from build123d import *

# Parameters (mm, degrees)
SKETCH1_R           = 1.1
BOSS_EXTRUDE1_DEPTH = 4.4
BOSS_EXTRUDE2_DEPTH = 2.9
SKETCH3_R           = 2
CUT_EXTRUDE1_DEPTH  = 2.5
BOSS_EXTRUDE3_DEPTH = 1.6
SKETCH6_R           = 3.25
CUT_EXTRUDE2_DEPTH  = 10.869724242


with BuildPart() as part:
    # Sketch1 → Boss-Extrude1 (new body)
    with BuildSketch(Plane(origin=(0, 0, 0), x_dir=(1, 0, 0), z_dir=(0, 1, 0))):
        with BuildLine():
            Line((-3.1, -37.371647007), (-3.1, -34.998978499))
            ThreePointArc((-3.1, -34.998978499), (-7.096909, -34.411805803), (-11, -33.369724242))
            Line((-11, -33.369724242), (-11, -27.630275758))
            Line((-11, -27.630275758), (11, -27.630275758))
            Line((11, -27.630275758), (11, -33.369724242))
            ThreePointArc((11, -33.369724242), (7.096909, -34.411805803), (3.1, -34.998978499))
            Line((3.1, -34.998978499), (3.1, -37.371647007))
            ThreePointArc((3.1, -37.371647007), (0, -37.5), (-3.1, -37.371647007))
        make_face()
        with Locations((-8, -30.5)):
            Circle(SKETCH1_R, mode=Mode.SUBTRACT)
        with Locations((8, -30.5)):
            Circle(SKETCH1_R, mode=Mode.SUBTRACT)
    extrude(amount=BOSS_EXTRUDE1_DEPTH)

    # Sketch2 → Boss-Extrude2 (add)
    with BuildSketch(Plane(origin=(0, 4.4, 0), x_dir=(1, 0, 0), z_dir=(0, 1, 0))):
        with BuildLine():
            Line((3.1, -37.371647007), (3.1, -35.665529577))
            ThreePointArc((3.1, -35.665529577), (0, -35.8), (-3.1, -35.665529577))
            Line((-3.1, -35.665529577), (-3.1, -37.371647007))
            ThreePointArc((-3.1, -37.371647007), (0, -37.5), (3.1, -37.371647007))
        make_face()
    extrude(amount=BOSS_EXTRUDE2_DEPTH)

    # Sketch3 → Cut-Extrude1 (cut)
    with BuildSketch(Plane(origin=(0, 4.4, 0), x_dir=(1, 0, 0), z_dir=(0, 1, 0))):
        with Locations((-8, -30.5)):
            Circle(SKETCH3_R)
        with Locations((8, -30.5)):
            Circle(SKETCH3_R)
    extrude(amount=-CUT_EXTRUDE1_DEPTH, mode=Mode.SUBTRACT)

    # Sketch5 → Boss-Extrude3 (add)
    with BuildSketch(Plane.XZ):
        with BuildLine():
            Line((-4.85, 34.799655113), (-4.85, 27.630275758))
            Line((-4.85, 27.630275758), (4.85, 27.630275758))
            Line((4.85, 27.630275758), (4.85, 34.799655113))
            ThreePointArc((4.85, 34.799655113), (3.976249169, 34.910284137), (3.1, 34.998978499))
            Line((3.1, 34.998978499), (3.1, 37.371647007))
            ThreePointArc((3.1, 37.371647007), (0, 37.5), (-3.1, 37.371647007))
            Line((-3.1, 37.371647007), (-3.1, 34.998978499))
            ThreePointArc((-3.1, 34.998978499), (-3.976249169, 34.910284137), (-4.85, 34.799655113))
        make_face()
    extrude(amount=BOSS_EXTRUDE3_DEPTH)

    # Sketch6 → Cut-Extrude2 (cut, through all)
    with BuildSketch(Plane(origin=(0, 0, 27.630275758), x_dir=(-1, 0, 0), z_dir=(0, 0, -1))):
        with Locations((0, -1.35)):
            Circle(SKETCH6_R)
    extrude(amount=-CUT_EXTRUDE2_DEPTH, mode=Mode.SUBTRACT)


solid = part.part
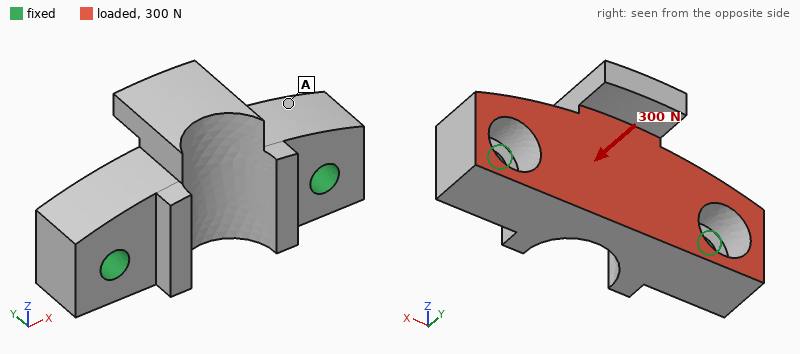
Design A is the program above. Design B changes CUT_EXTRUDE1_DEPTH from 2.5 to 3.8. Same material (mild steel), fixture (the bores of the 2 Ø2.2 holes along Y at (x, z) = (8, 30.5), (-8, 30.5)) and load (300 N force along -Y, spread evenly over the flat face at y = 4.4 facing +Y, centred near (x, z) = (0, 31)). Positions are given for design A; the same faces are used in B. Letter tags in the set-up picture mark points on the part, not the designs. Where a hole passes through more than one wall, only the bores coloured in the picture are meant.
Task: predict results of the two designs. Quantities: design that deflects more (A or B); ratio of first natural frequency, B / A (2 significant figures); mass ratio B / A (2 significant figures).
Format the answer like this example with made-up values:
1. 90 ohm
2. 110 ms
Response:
1. B
2. 0.45
3. 0.96
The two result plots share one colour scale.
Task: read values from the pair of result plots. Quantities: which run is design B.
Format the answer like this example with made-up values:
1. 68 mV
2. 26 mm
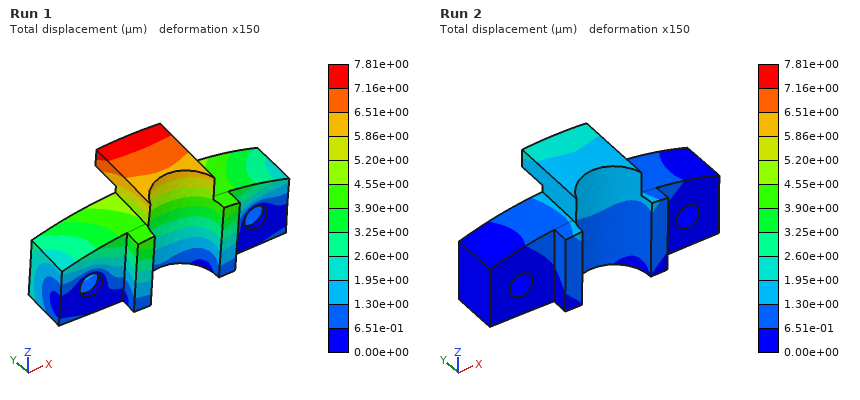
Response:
1. Run 1
